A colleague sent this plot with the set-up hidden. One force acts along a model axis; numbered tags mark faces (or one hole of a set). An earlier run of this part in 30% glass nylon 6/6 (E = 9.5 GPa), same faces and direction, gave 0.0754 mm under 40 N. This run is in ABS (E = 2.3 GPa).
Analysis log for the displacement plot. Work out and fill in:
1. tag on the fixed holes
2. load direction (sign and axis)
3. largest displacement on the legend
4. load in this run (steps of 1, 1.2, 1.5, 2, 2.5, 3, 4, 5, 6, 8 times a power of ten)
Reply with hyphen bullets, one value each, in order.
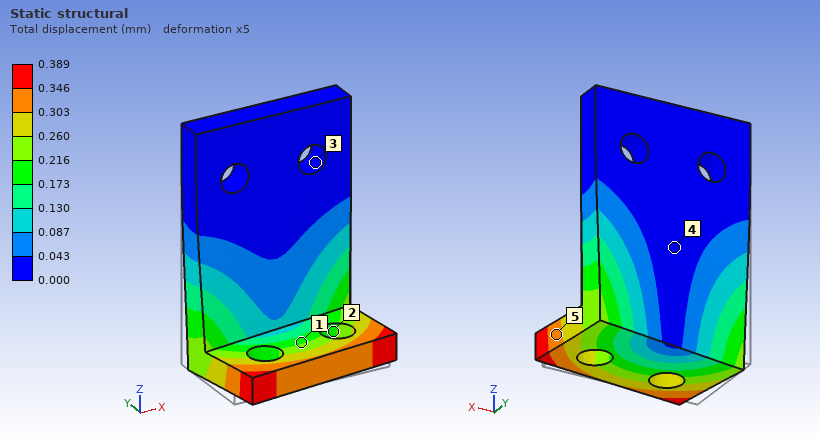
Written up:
- 3
- +X
- 0.389 mm
- 50 N
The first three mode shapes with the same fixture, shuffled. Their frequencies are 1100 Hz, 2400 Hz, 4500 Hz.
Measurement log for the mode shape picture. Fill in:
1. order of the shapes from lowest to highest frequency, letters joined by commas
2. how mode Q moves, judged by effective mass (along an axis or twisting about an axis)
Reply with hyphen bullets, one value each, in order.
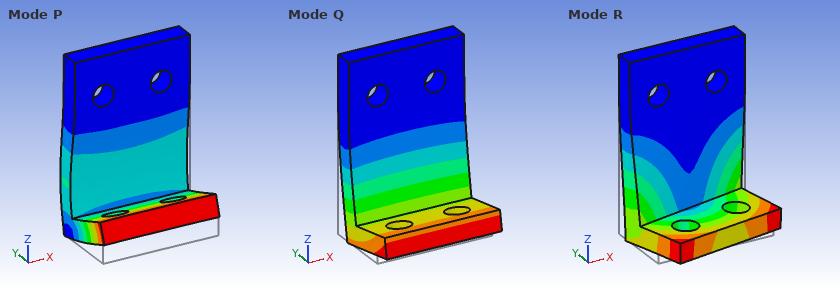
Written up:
- Q, R, P
- along Y
